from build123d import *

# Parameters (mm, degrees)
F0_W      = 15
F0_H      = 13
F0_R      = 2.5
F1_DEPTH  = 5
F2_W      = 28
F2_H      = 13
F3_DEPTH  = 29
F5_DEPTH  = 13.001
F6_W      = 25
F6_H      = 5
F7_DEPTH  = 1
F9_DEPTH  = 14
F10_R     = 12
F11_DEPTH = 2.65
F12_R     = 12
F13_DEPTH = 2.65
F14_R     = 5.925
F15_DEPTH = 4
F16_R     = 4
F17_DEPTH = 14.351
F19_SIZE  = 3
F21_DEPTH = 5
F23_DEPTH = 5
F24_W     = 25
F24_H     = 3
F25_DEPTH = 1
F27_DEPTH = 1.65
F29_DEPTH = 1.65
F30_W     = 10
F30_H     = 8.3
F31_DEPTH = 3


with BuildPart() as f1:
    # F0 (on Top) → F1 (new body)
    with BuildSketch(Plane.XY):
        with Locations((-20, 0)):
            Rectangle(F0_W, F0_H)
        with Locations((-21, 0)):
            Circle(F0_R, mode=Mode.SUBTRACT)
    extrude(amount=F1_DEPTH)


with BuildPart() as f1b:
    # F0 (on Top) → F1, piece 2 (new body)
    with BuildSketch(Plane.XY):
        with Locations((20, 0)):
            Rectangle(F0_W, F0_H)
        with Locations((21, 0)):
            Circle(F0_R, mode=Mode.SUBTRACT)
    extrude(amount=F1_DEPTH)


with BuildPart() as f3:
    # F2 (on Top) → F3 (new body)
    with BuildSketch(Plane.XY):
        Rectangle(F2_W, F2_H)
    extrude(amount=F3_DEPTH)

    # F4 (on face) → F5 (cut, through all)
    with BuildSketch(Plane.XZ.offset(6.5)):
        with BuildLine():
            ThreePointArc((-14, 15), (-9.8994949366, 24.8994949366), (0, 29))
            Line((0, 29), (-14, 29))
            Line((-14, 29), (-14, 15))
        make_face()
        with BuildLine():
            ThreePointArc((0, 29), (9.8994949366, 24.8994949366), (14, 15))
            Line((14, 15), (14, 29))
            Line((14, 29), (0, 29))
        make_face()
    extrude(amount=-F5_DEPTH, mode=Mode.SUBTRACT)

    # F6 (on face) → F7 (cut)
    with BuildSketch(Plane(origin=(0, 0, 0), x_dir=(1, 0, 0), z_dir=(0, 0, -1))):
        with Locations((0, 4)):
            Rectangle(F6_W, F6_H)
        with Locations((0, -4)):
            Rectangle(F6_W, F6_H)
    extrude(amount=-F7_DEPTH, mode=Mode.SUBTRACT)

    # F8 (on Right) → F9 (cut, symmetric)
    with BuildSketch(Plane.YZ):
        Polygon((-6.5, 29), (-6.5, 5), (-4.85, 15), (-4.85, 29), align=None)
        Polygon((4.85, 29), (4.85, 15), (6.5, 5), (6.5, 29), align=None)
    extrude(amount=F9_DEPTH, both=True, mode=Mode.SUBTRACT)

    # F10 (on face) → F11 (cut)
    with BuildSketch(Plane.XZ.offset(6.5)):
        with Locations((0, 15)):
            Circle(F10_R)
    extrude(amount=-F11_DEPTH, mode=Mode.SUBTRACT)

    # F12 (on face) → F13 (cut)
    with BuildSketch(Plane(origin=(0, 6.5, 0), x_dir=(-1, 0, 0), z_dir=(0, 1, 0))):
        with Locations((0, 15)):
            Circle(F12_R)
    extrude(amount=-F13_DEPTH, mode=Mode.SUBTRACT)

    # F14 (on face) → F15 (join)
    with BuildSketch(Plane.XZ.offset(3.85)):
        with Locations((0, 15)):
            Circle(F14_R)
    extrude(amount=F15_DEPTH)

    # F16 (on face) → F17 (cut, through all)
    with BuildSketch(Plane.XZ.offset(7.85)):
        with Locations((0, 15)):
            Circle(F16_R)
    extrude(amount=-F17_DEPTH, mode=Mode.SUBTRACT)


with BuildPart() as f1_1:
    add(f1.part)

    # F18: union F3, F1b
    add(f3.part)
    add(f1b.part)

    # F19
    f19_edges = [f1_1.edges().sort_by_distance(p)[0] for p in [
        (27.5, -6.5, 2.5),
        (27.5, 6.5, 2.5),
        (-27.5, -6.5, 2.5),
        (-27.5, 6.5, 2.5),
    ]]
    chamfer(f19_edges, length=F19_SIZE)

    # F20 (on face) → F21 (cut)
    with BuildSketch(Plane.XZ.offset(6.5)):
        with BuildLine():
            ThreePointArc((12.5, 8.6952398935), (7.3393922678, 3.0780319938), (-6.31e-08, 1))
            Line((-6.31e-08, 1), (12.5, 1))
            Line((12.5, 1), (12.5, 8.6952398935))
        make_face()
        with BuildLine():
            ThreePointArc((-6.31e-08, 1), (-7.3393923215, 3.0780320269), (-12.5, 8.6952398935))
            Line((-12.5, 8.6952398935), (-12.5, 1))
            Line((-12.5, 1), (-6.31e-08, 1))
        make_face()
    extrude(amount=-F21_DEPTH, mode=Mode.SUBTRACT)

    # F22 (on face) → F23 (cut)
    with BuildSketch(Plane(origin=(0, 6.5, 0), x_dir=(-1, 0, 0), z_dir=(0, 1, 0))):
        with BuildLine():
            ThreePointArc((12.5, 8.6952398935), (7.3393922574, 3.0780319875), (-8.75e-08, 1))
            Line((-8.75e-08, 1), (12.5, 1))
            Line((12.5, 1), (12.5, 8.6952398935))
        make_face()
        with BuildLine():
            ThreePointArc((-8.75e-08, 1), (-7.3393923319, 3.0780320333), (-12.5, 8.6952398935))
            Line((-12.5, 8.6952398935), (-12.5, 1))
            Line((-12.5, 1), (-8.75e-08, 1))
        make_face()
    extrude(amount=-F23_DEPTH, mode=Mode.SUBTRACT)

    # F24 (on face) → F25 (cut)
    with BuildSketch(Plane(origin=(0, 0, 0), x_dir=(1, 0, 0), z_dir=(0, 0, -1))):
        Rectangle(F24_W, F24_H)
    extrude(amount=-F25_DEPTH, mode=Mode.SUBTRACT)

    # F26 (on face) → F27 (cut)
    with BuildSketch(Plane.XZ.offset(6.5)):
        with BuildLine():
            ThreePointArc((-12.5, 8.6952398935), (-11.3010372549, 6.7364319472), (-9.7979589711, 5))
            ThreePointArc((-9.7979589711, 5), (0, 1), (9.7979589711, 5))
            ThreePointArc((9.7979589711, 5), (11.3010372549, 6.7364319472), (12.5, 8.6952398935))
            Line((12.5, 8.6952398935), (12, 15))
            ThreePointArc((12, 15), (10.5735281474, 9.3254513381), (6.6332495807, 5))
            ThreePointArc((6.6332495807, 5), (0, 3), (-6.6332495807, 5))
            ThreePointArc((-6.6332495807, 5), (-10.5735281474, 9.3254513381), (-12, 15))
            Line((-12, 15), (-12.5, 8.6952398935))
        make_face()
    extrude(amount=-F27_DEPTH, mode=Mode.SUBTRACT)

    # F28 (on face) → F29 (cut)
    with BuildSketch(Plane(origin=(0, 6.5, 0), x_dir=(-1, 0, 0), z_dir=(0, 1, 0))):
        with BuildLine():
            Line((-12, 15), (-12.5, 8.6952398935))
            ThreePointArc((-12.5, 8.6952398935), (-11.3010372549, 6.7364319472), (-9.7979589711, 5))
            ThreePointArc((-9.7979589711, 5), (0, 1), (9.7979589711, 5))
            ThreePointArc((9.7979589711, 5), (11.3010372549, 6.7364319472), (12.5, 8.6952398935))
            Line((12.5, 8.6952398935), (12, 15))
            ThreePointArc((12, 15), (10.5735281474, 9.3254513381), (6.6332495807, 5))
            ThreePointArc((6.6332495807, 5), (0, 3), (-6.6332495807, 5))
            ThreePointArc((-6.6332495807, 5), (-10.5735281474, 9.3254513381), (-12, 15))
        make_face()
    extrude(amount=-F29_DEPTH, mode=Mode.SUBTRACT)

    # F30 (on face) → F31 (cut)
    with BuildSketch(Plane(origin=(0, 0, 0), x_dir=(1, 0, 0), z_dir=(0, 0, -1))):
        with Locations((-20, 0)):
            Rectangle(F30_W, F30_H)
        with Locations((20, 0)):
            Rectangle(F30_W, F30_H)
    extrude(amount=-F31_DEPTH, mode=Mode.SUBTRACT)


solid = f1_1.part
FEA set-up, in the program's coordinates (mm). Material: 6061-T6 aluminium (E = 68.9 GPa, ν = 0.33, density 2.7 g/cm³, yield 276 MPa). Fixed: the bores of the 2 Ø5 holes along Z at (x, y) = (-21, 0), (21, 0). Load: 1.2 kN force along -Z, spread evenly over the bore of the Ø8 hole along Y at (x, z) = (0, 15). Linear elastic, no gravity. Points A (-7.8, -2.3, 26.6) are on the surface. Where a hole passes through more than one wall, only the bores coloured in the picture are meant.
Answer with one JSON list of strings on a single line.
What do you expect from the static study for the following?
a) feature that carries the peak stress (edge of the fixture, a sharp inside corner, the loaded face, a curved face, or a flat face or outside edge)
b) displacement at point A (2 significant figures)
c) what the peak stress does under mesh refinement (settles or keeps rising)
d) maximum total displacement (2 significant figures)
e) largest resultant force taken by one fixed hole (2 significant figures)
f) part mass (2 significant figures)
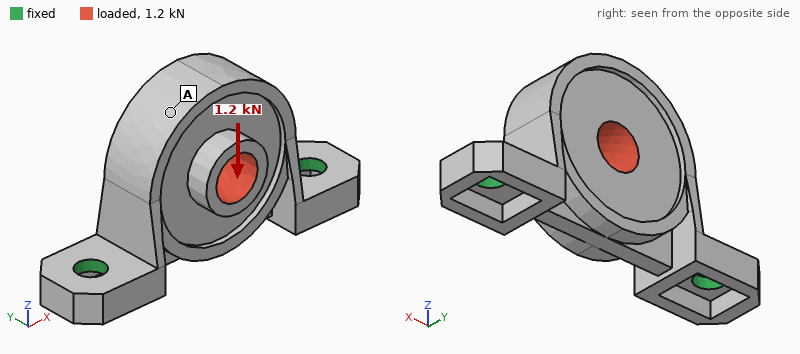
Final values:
["edge of the fixture", "72 µm", "keeps rising", "82 µm", "620 N", "18 g"]
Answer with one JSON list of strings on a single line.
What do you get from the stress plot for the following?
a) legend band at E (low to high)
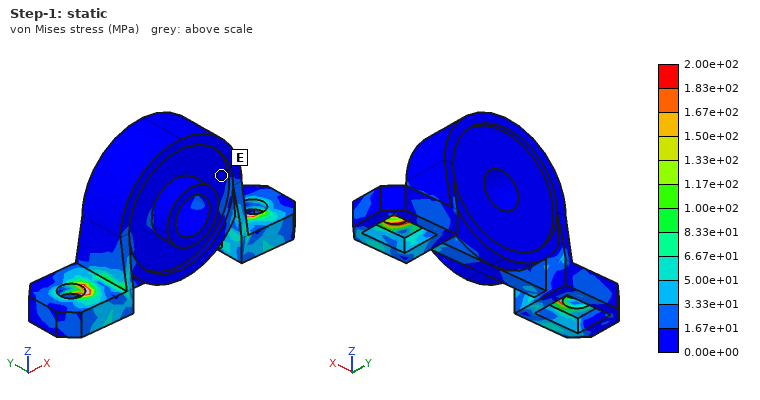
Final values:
["0.00e+00 to 1.67e+01 MPa"]
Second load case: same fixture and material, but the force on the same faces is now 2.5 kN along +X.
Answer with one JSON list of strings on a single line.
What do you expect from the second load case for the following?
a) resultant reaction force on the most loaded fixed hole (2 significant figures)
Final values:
["1.5 kN"]
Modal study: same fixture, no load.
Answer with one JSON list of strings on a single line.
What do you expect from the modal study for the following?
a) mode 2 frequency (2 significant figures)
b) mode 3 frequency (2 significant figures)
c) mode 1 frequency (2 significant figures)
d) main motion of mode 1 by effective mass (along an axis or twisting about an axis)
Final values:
["8800 Hz", "9100 Hz", "2900 Hz", "along Y"]
